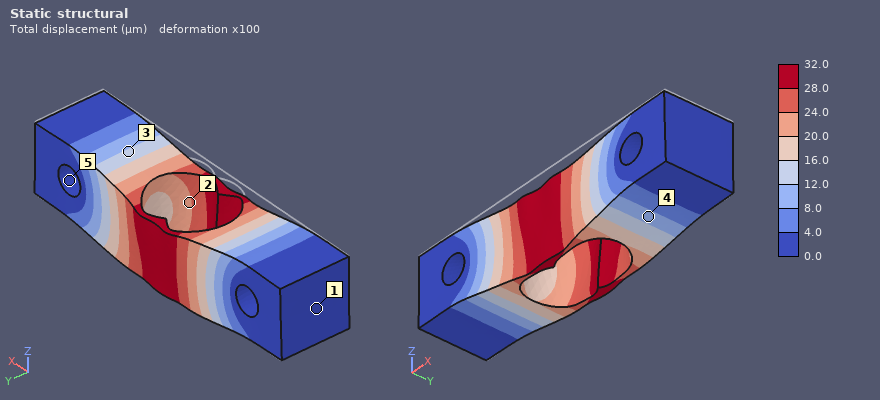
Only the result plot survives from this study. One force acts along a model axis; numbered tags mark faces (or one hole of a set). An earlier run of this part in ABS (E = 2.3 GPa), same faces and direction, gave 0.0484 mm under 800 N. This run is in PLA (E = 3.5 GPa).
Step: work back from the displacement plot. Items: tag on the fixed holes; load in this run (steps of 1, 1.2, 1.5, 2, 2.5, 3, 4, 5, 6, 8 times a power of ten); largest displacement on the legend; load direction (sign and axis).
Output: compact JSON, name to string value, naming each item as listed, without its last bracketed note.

{"tag on the fixed holes": "5", "load in this run": "800 N", "largest displacement on the legend": "32.0 µm", "load direction": "-Z"}
